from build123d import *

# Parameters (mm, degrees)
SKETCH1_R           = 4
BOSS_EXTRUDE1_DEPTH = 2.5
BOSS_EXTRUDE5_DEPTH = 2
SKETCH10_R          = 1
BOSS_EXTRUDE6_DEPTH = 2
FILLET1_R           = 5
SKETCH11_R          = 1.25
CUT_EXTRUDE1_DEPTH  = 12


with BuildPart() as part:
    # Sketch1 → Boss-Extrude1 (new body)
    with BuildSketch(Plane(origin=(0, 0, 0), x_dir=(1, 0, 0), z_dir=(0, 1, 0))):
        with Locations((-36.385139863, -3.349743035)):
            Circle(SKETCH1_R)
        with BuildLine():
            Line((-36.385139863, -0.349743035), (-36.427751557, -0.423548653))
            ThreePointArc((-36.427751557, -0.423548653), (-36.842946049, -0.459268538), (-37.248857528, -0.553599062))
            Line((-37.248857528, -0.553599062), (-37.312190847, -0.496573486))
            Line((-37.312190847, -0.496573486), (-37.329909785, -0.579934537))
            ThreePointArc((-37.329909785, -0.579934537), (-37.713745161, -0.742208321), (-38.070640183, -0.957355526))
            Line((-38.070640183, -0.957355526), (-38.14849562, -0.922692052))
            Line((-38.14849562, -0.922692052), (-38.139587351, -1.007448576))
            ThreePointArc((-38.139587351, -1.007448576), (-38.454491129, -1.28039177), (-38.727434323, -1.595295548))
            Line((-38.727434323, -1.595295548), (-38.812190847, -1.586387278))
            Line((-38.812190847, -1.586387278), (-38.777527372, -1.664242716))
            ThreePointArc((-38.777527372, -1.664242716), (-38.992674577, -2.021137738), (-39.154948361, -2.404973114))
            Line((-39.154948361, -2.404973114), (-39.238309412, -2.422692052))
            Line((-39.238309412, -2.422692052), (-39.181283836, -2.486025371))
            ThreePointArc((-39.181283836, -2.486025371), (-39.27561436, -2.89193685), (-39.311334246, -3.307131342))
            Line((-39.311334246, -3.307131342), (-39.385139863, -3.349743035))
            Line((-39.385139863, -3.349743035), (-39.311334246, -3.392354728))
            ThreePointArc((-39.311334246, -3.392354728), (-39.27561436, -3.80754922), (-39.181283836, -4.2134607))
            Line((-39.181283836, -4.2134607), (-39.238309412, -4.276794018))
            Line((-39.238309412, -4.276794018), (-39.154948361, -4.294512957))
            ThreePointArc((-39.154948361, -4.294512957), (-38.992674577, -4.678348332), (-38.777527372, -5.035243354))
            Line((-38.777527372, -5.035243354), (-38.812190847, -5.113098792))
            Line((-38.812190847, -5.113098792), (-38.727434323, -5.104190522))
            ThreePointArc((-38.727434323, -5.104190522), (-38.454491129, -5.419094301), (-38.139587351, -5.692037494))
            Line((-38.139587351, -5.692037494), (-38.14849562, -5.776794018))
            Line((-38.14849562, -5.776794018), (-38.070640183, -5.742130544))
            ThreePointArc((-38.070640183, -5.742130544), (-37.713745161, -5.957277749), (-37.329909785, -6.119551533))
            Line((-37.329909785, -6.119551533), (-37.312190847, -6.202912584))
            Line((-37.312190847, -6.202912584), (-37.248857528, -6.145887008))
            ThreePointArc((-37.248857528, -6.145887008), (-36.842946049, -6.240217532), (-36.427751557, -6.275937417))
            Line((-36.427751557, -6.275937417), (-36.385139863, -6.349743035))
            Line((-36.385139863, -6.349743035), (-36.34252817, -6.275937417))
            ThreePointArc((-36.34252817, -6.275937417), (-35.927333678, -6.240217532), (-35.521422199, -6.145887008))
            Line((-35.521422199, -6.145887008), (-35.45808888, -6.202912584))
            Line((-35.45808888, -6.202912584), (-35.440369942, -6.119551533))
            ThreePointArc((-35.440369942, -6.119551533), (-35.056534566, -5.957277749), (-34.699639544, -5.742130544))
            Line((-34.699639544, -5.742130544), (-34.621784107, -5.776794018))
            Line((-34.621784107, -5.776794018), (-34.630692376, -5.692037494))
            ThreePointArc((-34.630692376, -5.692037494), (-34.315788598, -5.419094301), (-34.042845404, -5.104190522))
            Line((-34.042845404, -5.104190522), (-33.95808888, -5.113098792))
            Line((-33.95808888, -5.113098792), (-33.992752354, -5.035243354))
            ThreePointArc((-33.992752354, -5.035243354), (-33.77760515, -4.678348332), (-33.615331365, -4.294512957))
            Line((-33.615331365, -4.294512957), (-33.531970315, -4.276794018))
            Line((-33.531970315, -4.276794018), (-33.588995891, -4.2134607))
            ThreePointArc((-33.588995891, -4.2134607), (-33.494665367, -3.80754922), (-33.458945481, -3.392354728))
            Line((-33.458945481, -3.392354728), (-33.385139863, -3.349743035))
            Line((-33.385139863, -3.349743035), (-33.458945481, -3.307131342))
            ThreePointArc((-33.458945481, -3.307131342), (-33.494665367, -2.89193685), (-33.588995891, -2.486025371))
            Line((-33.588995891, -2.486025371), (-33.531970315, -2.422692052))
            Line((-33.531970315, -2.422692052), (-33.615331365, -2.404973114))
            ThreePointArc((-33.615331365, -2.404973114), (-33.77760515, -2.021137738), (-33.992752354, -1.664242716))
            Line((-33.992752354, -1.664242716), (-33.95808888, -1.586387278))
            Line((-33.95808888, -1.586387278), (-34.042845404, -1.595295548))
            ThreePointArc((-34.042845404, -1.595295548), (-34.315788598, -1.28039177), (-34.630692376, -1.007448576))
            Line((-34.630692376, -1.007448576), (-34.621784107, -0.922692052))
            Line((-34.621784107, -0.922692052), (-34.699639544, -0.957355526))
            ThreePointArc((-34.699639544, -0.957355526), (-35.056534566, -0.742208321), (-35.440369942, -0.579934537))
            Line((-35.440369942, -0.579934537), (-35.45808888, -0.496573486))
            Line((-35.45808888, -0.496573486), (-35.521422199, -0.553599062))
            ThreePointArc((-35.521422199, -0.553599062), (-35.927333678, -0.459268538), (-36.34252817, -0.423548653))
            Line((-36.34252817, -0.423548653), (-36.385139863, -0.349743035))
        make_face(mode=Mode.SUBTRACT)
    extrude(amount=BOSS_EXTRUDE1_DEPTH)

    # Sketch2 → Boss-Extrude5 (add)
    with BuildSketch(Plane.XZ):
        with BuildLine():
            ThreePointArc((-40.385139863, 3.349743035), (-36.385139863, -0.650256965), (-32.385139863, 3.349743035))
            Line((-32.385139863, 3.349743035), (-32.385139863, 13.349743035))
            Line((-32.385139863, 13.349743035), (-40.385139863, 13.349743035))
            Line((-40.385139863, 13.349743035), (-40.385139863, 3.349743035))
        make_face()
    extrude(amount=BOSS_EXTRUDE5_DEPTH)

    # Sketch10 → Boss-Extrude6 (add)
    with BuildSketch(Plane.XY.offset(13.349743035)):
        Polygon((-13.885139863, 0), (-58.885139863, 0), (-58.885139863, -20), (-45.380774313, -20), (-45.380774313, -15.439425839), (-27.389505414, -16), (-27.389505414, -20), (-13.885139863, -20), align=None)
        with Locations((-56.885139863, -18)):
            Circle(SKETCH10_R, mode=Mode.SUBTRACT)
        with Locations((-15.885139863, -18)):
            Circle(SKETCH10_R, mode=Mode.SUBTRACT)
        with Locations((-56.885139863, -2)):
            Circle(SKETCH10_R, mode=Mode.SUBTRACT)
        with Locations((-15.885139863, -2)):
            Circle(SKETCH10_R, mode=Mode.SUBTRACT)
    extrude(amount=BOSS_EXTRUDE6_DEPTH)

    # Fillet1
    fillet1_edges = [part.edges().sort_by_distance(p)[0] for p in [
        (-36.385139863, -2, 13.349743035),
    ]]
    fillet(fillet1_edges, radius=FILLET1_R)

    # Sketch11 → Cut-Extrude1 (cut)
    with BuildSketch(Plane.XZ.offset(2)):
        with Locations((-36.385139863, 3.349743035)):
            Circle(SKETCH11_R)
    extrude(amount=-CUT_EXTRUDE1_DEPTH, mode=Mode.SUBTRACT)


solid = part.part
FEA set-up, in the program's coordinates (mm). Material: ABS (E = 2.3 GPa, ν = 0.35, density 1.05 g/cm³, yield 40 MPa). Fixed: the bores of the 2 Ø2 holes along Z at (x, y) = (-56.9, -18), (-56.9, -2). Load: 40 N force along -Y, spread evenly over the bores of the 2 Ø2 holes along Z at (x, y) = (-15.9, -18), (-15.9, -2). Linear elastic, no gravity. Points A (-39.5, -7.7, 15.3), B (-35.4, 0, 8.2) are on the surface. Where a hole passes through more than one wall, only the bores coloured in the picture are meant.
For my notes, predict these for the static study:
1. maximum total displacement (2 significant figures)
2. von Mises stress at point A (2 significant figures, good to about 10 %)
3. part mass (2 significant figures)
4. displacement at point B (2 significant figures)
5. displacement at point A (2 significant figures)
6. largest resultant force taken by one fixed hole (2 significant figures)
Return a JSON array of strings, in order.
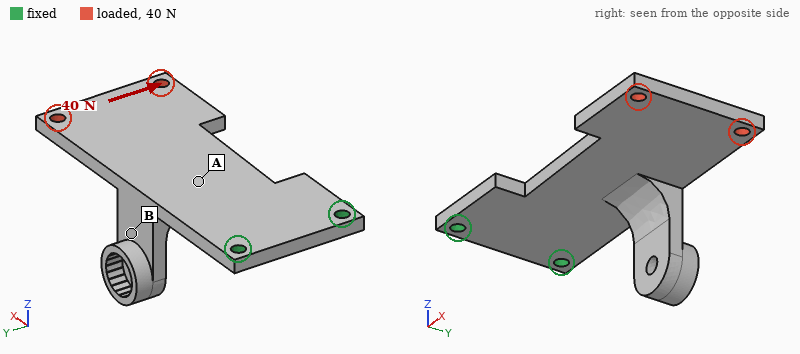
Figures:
["0.63 mm", "4.4 MPa", "2.0 g", "0.19 mm", "0.11 mm", "100 N"]
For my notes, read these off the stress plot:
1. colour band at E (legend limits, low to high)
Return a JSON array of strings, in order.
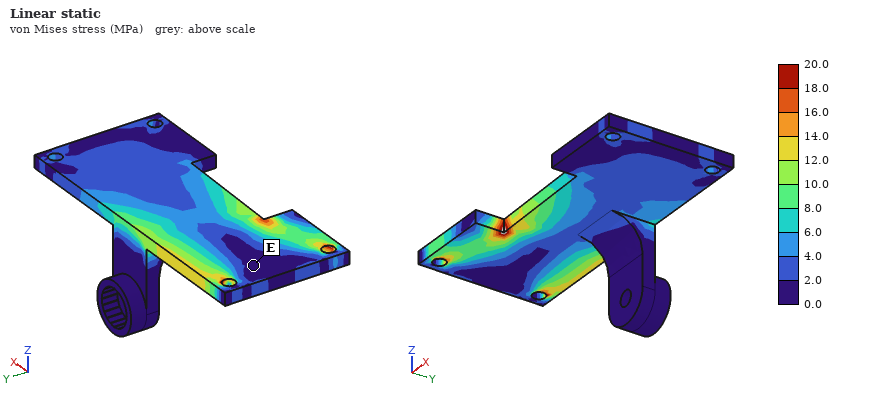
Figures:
["0.0 to 2.0 MPa"]
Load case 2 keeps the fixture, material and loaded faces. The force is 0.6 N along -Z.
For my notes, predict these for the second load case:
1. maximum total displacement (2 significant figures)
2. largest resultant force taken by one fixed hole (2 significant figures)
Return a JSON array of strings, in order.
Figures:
["0.56 mm", "0.30 N"]
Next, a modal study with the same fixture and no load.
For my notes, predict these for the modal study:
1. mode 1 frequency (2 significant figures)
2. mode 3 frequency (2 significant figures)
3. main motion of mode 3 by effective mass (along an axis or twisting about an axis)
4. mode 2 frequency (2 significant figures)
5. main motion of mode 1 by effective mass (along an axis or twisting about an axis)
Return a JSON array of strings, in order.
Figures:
["230 Hz", "1500 Hz", "along Z", "880 Hz", "along Z"]
